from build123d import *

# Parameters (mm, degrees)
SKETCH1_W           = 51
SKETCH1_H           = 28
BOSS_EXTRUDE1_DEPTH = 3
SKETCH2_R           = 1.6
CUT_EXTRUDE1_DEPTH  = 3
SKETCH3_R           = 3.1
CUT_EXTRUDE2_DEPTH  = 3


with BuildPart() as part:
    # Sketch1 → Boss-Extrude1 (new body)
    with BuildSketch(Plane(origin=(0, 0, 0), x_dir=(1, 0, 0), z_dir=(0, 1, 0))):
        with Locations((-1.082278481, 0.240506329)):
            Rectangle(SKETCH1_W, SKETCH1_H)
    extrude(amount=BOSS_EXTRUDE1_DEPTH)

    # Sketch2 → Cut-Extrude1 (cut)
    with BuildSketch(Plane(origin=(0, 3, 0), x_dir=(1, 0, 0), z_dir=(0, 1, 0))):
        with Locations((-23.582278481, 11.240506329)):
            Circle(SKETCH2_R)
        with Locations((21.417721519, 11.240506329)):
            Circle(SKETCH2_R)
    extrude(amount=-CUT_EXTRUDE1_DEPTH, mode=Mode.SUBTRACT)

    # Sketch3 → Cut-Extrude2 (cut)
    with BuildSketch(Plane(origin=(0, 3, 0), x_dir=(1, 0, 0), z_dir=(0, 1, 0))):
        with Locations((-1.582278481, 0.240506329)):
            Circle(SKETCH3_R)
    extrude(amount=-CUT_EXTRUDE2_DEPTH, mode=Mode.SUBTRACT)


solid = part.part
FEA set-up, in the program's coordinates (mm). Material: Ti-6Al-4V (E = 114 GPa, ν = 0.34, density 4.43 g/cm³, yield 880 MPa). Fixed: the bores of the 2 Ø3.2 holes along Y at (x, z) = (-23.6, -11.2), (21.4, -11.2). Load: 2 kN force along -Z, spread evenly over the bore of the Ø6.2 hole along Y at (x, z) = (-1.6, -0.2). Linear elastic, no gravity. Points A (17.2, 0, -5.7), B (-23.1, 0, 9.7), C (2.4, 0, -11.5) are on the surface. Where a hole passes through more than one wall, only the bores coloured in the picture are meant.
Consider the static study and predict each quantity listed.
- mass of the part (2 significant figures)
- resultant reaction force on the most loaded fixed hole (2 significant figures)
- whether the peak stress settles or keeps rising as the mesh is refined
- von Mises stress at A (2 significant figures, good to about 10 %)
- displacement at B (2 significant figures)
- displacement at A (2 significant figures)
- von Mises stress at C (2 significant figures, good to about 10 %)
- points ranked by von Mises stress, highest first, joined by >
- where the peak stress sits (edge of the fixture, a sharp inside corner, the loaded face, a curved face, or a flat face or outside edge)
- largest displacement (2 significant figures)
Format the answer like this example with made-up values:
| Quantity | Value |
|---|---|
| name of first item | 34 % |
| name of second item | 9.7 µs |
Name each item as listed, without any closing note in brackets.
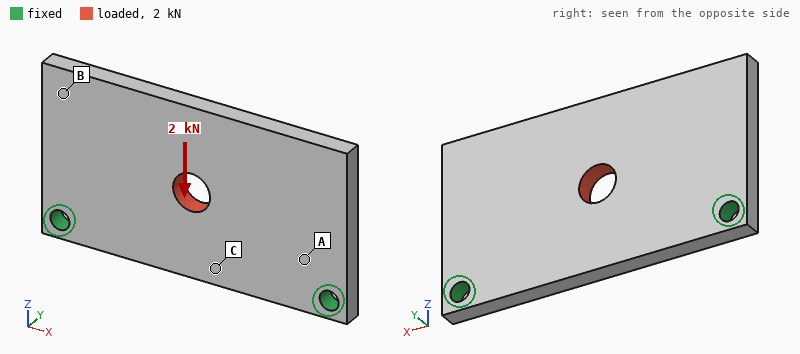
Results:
| Quantity | Value |
|---|---|
| mass of the part | 18 g |
| resultant reaction force on the most loaded fixed hole | 1.2 kN |
| whether the peak stress settles or keeps rising as the mesh is refined | keeps rising |
| von Mises stress at A | 37 MPa |
| displacement at B | 4.4 µm |
| displacement at A | 3.2 µm |
| von Mises stress at C | 20 MPa |
| points ranked by von Mises stress, highest first, joined by > | A > C > B |
| where the peak stress sits | edge of the fixture |
| largest displacement | 13 µm |
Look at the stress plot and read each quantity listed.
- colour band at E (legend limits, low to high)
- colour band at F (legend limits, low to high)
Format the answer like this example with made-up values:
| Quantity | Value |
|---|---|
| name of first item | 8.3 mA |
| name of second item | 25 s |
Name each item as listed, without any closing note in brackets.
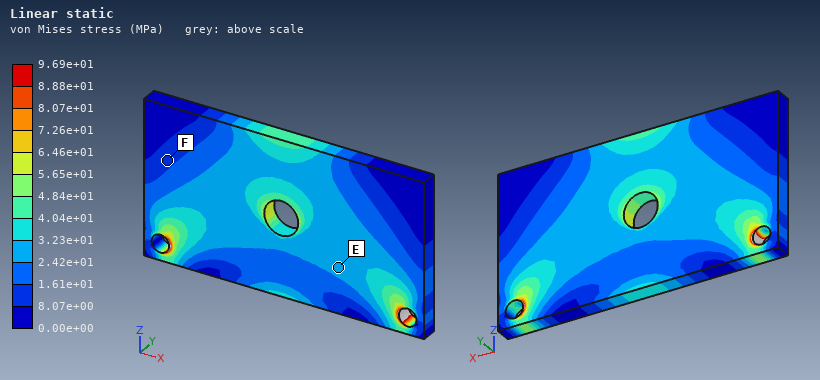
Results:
| Quantity | Value |
|---|---|
| colour band at E | 2.42e+01 to 3.23e+01 MPa |
| colour band at F | 8.07e+00 to 1.61e+01 MPa |
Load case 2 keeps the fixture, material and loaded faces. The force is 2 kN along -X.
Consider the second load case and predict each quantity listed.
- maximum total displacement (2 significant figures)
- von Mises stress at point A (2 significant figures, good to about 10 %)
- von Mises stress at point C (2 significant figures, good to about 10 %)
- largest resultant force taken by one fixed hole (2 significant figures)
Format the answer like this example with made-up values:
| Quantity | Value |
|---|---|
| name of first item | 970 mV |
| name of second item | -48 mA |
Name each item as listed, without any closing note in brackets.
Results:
| Quantity | Value |
|---|---|
| maximum total displacement | 8.7 µm |
| von Mises stress at point A | 29 MPa |
| von Mises stress at point C | 11 MPa |
| largest resultant force taken by one fixed hole | 1.1 kN |
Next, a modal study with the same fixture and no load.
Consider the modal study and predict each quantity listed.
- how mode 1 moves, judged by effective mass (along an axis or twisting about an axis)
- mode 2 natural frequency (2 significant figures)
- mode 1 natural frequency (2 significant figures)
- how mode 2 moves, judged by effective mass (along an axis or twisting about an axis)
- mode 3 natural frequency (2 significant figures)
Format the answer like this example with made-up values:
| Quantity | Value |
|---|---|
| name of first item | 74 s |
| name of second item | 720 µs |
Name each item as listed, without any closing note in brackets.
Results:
| Quantity | Value |
|---|---|
| how mode 1 moves, judged by effective mass | along Y |
| mode 2 natural frequency | 5700 Hz |
| mode 1 natural frequency | 2700 Hz |
| how mode 2 moves, judged by effective mass | twisting about Z |
| mode 3 natural frequency | 7600 Hz |
